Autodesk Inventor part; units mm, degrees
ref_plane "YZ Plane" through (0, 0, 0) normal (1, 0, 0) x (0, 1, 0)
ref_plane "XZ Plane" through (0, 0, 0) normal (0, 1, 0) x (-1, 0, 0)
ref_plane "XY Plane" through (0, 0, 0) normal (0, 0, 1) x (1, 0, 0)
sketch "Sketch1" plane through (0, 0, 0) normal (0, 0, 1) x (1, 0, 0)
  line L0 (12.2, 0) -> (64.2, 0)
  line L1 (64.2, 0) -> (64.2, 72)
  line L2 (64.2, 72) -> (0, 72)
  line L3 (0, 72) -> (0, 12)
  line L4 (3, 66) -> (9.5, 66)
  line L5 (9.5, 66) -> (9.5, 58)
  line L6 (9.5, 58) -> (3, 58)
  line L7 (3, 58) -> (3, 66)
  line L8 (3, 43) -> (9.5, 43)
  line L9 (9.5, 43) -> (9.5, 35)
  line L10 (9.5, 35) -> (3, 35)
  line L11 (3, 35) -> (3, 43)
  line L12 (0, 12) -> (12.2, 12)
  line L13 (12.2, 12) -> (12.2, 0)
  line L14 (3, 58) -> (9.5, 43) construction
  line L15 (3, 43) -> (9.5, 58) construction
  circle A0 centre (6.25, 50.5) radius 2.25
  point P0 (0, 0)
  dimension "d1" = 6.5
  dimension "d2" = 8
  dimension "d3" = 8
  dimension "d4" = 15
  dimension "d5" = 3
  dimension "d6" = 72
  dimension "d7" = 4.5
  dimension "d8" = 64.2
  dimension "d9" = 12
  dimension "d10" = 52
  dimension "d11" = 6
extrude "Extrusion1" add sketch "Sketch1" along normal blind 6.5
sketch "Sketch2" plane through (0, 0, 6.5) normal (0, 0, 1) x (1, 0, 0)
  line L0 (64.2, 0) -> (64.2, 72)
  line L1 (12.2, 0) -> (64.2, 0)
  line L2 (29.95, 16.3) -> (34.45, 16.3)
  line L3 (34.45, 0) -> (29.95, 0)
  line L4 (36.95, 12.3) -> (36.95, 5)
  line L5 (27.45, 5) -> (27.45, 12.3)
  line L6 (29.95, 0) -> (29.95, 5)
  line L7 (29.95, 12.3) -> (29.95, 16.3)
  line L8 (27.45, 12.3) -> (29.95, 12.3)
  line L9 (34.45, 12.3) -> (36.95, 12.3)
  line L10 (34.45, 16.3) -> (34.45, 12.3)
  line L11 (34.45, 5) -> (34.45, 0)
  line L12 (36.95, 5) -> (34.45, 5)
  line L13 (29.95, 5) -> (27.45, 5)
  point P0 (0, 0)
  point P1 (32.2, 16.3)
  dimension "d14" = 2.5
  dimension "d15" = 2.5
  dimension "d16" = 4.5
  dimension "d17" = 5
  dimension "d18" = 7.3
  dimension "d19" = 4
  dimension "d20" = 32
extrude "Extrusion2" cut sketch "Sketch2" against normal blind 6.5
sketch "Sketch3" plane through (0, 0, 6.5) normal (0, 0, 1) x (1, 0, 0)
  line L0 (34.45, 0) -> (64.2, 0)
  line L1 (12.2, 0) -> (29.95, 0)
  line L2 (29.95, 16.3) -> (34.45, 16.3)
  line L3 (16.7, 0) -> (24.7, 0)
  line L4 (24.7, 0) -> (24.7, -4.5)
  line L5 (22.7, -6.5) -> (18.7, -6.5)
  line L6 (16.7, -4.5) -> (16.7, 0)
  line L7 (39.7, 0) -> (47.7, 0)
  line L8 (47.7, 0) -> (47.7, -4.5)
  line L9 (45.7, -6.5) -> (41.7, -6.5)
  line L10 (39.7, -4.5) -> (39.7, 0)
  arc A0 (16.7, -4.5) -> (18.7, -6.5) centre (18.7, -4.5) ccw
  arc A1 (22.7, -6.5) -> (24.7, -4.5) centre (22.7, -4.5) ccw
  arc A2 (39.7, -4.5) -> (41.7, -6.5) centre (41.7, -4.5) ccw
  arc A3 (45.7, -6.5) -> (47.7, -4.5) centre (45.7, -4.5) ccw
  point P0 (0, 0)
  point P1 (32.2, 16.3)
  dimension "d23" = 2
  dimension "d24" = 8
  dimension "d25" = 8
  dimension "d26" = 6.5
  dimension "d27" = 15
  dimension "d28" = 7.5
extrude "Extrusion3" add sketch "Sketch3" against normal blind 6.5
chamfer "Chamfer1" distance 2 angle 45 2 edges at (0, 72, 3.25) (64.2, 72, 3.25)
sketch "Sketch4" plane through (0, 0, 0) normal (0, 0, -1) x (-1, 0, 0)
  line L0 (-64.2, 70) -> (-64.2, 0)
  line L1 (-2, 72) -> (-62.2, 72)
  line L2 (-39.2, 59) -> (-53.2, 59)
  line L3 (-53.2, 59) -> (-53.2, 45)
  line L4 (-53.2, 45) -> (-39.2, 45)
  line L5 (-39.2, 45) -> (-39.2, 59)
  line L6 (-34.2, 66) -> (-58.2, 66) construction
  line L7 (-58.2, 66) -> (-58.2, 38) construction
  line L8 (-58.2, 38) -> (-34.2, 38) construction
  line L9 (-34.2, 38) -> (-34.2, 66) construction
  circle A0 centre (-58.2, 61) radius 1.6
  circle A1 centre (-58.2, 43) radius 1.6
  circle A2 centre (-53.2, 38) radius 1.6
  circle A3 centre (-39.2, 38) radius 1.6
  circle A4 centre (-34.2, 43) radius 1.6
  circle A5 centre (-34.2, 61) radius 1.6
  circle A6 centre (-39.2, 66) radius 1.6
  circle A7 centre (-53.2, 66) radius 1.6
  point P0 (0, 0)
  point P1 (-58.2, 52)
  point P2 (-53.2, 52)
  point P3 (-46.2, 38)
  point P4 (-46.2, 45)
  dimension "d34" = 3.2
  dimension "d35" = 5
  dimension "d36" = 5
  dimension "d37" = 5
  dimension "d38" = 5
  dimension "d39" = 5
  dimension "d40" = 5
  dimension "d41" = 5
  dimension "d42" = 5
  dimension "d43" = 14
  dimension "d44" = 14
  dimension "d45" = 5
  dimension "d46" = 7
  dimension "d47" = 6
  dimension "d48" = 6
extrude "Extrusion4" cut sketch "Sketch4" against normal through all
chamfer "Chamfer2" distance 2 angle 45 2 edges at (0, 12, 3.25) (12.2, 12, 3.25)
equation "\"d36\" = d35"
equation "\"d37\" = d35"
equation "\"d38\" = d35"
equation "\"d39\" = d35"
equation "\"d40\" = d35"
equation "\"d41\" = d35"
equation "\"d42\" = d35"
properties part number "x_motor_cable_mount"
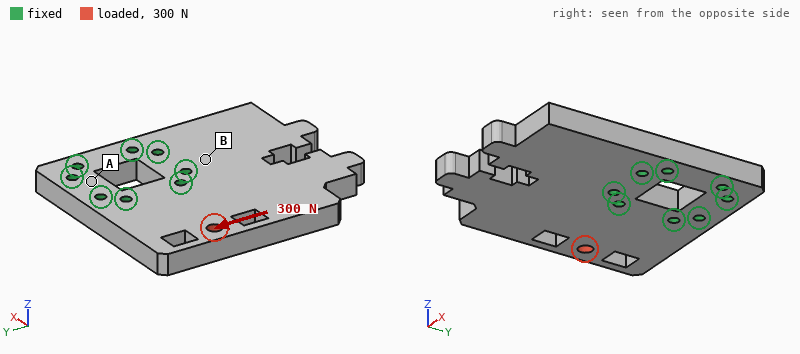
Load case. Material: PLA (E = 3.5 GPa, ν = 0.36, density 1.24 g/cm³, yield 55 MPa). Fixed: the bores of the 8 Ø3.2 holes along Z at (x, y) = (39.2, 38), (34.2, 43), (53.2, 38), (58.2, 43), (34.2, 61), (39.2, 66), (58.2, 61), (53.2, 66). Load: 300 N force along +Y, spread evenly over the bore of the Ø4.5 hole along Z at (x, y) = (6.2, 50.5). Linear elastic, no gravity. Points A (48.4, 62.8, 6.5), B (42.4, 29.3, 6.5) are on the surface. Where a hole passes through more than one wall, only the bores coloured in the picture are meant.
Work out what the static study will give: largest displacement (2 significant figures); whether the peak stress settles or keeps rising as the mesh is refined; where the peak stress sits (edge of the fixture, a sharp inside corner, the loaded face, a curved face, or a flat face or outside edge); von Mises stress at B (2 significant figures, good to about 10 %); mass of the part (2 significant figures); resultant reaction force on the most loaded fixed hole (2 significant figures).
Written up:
60 µm
keeps rising
edge of the fixture
1.7 MPa
33 g
190 N
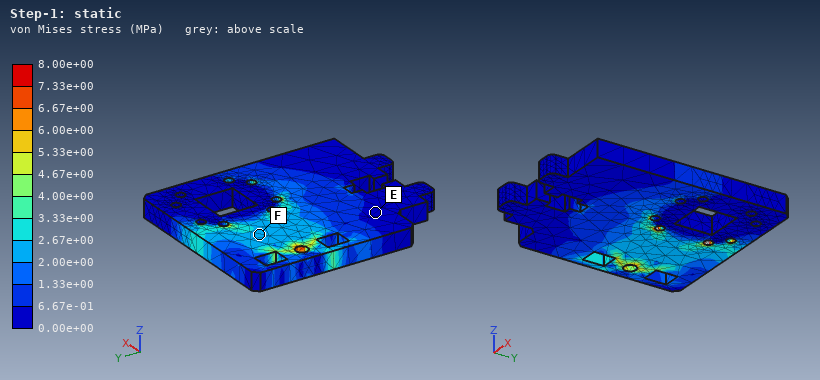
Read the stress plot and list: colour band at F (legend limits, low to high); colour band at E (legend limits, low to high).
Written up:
2.00e+00 to 2.67e+00 MPa
0.00e+00 to 6.67e-01 MPa
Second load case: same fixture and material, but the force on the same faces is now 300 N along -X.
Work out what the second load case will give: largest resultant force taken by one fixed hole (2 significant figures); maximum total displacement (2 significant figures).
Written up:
110 N
24 µm
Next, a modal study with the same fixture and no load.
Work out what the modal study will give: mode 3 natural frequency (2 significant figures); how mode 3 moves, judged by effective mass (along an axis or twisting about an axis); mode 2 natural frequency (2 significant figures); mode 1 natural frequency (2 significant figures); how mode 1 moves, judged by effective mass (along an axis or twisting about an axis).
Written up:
1700 Hz
along Z
1300 Hz
950 Hz
along Z
